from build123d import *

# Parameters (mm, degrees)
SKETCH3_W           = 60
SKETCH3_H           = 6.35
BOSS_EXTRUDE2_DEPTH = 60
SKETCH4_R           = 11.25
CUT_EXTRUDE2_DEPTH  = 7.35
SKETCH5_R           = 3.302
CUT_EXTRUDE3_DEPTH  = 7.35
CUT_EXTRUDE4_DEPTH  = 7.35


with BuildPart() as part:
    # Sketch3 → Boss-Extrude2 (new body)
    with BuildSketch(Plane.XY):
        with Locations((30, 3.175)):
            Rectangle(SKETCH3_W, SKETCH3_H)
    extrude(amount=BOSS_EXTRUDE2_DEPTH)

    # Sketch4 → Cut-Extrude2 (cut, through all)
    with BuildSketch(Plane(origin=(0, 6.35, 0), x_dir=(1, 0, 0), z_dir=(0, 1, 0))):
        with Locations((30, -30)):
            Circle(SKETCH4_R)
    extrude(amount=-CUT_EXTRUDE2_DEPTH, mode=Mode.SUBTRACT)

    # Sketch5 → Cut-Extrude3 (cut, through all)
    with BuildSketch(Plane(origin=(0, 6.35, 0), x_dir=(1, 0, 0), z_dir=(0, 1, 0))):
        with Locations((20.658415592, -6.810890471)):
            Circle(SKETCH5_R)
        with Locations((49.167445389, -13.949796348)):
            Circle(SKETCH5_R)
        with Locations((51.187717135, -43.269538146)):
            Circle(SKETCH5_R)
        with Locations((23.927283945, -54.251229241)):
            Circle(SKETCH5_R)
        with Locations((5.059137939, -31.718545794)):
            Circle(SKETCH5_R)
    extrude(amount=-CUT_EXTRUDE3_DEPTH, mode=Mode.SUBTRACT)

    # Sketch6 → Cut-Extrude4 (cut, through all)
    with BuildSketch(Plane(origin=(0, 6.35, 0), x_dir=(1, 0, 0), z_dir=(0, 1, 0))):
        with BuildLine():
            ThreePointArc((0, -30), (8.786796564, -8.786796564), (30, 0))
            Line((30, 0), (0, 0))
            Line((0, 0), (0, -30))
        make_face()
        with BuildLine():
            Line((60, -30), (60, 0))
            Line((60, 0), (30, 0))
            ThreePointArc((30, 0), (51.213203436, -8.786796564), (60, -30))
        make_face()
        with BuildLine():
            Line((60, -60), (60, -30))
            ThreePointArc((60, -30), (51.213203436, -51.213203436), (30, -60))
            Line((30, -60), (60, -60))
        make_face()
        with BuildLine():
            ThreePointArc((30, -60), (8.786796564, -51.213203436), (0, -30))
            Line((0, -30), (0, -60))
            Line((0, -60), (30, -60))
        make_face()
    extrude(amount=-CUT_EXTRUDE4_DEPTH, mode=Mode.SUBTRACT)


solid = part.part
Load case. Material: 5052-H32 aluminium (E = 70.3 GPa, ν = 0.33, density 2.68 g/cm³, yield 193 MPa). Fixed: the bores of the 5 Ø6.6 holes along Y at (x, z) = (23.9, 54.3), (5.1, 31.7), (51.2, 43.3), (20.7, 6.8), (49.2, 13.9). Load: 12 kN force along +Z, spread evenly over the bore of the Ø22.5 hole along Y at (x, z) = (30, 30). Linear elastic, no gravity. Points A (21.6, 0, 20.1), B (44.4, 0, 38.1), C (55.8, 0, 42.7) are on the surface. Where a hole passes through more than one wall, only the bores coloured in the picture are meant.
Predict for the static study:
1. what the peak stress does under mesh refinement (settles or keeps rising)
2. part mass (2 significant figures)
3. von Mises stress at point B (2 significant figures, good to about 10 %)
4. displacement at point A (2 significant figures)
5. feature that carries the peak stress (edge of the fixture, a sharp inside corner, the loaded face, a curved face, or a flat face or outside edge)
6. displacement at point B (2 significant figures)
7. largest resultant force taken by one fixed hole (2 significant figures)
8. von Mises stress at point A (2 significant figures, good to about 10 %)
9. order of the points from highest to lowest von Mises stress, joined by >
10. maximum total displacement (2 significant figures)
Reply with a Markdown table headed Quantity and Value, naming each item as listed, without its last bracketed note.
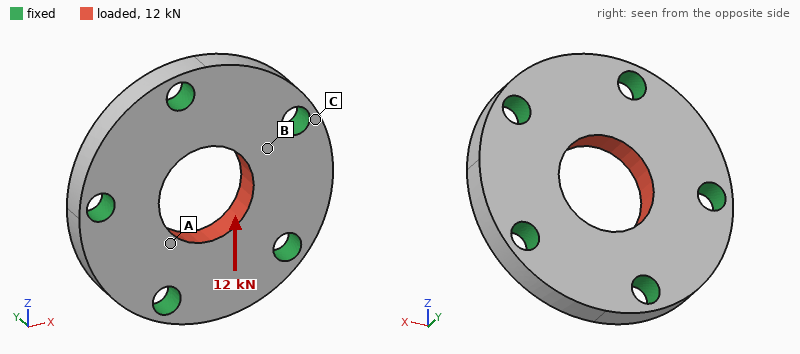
| Quantity | Value |
|---|---|
| what the peak stress does under mesh refinement | keeps rising |
| part mass | 38 g |
| von Mises stress at point B | 25 MPa |
| displacement at point A | 5.2 µm |
| feature that carries the peak stress | edge of the fixture |
| displacement at point B | 3.2 µm |
| largest resultant force taken by one fixed hole | 3.2 kN |
| von Mises stress at point A | 38 MPa |
| order of the points from highest to lowest von Mises stress, joined by > | A > B > C |
| maximum total displacement | 7.8 µm |
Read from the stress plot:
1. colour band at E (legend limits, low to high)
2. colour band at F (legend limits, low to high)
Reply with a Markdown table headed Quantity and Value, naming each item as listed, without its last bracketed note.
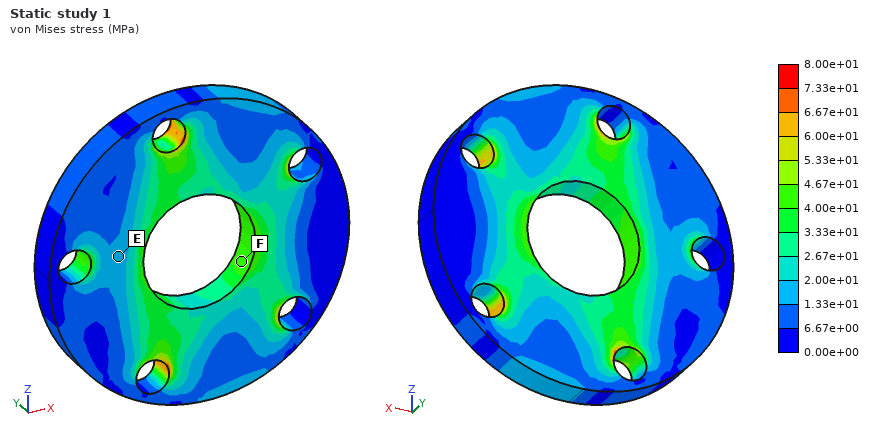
| Quantity | Value |
|---|---|
| colour band at E | 1.33e+01 to 2.00e+01 MPa |
| colour band at F | 4.00e+01 to 4.67e+01 MPa |
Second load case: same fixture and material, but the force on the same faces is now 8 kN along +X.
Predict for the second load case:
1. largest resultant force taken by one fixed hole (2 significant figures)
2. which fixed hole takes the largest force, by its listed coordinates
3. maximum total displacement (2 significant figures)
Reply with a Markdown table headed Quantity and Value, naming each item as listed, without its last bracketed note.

| Quantity | Value |
|---|---|
| largest resultant force taken by one fixed hole | 2.2 kN |
| which fixed hole takes the largest force, by its listed coordinates | (5.1, 31.7) |
| maximum total displacement | 5.2 µm |
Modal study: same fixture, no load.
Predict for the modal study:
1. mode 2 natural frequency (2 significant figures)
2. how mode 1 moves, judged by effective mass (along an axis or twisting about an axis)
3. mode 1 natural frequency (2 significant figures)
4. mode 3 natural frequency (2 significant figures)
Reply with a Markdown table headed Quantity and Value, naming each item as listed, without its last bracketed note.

| Quantity | Value |
|---|---|
| mode 2 natural frequency | 34 kHz |
| how mode 1 moves, judged by effective mass | along Y |
| mode 1 natural frequency | 30 kHz |
| mode 3 natural frequency | 34 kHz |
